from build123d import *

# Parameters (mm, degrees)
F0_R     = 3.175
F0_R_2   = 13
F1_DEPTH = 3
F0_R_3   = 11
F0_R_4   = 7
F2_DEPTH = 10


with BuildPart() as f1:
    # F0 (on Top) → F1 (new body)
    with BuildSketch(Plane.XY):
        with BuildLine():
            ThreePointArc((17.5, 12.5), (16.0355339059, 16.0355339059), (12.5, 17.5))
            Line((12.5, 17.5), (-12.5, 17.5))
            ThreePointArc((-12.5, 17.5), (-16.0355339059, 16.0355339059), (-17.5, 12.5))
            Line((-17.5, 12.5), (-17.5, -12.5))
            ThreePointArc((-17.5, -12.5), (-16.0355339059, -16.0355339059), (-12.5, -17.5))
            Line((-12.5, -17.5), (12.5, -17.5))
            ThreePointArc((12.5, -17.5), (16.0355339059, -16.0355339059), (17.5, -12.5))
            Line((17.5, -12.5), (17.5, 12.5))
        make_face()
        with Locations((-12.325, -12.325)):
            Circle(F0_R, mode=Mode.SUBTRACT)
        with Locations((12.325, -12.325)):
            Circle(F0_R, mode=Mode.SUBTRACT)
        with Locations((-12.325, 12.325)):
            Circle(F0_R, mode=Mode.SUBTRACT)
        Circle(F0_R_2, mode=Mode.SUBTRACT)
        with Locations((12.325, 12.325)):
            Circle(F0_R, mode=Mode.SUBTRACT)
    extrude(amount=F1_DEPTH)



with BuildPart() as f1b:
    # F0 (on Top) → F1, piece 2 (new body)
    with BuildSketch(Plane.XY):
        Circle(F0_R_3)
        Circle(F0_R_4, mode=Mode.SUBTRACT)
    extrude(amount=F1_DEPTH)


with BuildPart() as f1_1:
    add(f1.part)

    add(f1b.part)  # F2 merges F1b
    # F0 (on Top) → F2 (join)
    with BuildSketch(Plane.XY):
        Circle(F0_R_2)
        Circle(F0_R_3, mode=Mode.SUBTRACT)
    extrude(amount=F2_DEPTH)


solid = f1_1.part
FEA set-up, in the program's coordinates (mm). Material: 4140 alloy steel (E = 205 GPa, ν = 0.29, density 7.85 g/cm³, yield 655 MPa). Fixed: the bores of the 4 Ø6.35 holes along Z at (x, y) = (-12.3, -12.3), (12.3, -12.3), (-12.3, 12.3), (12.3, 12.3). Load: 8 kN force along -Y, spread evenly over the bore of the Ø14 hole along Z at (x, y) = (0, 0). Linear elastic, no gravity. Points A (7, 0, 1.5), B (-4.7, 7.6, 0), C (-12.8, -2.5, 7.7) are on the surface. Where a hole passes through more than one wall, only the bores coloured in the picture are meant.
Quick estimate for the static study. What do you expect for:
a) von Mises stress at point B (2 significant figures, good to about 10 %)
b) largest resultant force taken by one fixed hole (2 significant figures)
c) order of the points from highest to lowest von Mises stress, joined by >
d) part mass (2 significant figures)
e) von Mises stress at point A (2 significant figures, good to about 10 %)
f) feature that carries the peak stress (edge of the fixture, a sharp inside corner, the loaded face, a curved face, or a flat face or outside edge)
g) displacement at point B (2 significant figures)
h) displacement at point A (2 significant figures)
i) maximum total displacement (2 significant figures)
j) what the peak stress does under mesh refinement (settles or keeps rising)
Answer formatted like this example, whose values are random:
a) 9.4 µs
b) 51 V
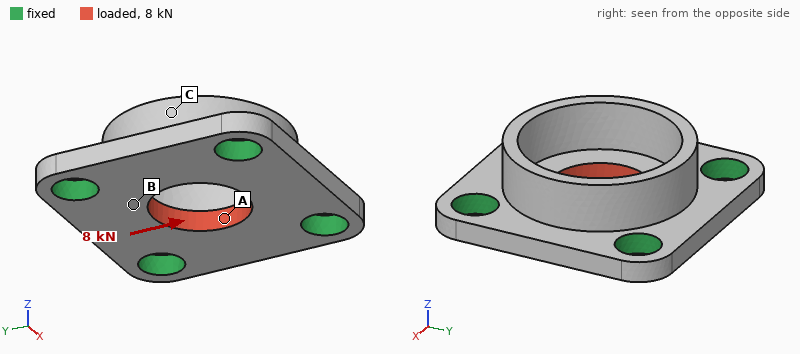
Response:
a) 59 MPa
b) 2.1 kN
c) A > B > C
d) 30 g
e) 100 MPa
f) edge of the fixture
g) 3.4 µm
h) 3.2 µm
i) 5.2 µm
j) keeps rising
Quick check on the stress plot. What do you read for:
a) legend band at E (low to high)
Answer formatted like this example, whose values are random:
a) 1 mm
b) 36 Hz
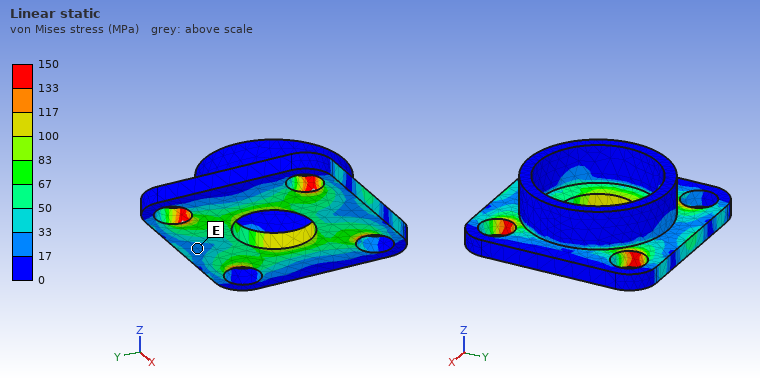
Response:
a) 17 to 33 MPa
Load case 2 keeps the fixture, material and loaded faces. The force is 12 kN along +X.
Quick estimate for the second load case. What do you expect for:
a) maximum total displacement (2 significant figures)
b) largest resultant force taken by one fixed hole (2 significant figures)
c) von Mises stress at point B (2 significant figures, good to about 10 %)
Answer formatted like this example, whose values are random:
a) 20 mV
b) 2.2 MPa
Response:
a) 7.8 µm
b) 3.2 kN
c) 110 MPa
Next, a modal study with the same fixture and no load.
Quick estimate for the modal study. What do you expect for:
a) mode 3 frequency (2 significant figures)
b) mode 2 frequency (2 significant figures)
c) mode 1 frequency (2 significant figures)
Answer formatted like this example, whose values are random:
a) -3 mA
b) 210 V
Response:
a) 35 kHz
b) 35 kHz
c) 29 kHz
